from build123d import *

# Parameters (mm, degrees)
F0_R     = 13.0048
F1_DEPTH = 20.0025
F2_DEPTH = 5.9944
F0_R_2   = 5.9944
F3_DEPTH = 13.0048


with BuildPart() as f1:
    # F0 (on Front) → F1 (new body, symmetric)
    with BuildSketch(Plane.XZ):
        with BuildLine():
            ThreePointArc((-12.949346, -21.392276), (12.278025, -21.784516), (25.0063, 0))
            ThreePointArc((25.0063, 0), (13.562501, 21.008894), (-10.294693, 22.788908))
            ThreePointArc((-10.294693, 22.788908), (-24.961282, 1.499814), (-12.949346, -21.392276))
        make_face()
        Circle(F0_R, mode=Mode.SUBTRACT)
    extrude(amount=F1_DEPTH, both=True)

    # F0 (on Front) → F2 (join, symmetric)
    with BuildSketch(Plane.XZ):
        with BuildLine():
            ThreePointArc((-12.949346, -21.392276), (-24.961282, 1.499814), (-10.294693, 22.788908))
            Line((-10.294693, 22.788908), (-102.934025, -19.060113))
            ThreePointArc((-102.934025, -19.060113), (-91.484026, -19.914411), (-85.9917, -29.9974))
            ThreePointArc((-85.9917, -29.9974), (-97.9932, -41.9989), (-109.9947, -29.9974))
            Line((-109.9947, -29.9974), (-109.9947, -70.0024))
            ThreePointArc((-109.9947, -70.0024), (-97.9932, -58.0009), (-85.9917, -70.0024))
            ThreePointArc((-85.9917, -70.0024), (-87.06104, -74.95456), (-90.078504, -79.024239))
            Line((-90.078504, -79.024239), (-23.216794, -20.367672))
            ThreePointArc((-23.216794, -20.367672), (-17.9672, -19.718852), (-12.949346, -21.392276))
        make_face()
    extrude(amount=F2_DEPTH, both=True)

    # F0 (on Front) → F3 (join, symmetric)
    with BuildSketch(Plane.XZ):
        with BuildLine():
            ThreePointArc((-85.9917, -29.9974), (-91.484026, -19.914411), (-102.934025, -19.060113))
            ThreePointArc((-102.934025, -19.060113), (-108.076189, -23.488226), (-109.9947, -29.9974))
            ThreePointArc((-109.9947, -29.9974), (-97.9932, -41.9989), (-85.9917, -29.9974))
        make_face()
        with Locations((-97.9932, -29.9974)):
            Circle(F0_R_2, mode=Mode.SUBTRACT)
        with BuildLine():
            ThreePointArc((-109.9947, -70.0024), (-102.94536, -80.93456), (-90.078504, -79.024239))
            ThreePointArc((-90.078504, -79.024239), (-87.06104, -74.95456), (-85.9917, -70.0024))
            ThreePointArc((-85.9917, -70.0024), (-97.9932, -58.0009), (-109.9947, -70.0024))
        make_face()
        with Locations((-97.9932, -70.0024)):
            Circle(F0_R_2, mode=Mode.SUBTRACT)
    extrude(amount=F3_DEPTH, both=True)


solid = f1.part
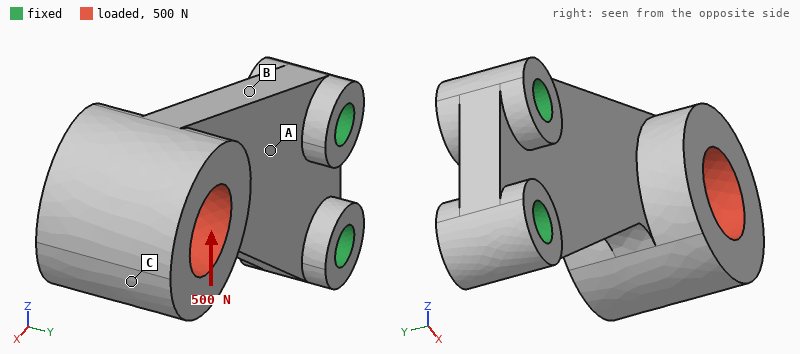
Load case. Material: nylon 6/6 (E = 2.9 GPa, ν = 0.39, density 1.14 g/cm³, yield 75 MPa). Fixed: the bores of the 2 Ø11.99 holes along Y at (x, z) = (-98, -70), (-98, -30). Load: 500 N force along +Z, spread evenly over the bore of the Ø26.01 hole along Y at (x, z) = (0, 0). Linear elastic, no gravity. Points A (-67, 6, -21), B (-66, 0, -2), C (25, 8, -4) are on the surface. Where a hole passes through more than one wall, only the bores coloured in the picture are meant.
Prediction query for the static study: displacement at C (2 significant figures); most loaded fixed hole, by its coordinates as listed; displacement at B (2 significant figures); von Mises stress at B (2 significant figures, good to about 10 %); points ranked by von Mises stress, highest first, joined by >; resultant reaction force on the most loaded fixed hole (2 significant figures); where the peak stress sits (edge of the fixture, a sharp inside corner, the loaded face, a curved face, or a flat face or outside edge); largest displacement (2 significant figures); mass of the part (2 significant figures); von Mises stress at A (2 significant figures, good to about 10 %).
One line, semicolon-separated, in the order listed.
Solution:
0.95 mm; (-98, -70); 0.17 mm; 7.3 MPa; B > A > C; 1.2 kN; a curved face; 0.97 mm; 140 g; 1.9 MPa
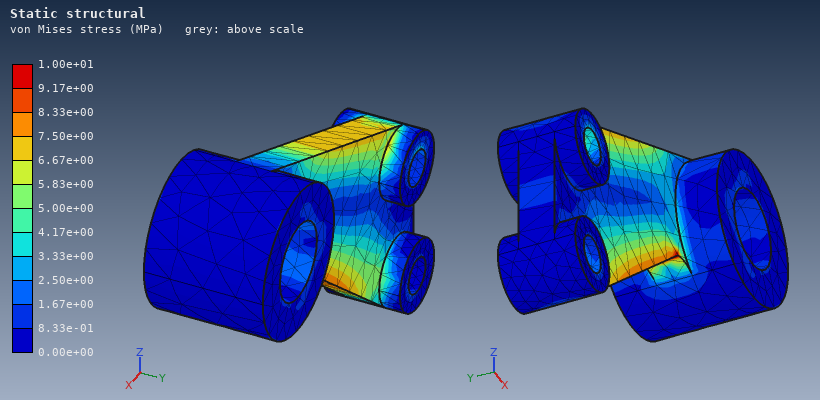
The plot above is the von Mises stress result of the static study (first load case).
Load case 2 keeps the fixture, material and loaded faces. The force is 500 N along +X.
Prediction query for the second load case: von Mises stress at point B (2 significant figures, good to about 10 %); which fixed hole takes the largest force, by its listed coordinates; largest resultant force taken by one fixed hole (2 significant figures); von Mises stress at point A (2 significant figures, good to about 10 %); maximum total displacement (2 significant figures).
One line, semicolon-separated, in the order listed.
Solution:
3.7 MPa; (-98, -30); 790 N; 1.9 MPa; 0.34 mm
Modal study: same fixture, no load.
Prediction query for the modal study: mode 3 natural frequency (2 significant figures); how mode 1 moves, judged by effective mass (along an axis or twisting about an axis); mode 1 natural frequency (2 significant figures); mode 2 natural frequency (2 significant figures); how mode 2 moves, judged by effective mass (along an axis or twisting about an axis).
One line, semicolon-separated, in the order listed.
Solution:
570 Hz; along Y; 150 Hz; 480 Hz; along Z
